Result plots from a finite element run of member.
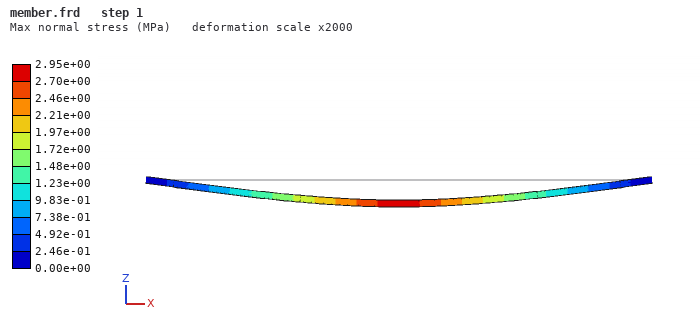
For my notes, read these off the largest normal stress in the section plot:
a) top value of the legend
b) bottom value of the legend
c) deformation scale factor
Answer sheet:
2.95e+00 MPa
0.00e+00 MPa
2000
